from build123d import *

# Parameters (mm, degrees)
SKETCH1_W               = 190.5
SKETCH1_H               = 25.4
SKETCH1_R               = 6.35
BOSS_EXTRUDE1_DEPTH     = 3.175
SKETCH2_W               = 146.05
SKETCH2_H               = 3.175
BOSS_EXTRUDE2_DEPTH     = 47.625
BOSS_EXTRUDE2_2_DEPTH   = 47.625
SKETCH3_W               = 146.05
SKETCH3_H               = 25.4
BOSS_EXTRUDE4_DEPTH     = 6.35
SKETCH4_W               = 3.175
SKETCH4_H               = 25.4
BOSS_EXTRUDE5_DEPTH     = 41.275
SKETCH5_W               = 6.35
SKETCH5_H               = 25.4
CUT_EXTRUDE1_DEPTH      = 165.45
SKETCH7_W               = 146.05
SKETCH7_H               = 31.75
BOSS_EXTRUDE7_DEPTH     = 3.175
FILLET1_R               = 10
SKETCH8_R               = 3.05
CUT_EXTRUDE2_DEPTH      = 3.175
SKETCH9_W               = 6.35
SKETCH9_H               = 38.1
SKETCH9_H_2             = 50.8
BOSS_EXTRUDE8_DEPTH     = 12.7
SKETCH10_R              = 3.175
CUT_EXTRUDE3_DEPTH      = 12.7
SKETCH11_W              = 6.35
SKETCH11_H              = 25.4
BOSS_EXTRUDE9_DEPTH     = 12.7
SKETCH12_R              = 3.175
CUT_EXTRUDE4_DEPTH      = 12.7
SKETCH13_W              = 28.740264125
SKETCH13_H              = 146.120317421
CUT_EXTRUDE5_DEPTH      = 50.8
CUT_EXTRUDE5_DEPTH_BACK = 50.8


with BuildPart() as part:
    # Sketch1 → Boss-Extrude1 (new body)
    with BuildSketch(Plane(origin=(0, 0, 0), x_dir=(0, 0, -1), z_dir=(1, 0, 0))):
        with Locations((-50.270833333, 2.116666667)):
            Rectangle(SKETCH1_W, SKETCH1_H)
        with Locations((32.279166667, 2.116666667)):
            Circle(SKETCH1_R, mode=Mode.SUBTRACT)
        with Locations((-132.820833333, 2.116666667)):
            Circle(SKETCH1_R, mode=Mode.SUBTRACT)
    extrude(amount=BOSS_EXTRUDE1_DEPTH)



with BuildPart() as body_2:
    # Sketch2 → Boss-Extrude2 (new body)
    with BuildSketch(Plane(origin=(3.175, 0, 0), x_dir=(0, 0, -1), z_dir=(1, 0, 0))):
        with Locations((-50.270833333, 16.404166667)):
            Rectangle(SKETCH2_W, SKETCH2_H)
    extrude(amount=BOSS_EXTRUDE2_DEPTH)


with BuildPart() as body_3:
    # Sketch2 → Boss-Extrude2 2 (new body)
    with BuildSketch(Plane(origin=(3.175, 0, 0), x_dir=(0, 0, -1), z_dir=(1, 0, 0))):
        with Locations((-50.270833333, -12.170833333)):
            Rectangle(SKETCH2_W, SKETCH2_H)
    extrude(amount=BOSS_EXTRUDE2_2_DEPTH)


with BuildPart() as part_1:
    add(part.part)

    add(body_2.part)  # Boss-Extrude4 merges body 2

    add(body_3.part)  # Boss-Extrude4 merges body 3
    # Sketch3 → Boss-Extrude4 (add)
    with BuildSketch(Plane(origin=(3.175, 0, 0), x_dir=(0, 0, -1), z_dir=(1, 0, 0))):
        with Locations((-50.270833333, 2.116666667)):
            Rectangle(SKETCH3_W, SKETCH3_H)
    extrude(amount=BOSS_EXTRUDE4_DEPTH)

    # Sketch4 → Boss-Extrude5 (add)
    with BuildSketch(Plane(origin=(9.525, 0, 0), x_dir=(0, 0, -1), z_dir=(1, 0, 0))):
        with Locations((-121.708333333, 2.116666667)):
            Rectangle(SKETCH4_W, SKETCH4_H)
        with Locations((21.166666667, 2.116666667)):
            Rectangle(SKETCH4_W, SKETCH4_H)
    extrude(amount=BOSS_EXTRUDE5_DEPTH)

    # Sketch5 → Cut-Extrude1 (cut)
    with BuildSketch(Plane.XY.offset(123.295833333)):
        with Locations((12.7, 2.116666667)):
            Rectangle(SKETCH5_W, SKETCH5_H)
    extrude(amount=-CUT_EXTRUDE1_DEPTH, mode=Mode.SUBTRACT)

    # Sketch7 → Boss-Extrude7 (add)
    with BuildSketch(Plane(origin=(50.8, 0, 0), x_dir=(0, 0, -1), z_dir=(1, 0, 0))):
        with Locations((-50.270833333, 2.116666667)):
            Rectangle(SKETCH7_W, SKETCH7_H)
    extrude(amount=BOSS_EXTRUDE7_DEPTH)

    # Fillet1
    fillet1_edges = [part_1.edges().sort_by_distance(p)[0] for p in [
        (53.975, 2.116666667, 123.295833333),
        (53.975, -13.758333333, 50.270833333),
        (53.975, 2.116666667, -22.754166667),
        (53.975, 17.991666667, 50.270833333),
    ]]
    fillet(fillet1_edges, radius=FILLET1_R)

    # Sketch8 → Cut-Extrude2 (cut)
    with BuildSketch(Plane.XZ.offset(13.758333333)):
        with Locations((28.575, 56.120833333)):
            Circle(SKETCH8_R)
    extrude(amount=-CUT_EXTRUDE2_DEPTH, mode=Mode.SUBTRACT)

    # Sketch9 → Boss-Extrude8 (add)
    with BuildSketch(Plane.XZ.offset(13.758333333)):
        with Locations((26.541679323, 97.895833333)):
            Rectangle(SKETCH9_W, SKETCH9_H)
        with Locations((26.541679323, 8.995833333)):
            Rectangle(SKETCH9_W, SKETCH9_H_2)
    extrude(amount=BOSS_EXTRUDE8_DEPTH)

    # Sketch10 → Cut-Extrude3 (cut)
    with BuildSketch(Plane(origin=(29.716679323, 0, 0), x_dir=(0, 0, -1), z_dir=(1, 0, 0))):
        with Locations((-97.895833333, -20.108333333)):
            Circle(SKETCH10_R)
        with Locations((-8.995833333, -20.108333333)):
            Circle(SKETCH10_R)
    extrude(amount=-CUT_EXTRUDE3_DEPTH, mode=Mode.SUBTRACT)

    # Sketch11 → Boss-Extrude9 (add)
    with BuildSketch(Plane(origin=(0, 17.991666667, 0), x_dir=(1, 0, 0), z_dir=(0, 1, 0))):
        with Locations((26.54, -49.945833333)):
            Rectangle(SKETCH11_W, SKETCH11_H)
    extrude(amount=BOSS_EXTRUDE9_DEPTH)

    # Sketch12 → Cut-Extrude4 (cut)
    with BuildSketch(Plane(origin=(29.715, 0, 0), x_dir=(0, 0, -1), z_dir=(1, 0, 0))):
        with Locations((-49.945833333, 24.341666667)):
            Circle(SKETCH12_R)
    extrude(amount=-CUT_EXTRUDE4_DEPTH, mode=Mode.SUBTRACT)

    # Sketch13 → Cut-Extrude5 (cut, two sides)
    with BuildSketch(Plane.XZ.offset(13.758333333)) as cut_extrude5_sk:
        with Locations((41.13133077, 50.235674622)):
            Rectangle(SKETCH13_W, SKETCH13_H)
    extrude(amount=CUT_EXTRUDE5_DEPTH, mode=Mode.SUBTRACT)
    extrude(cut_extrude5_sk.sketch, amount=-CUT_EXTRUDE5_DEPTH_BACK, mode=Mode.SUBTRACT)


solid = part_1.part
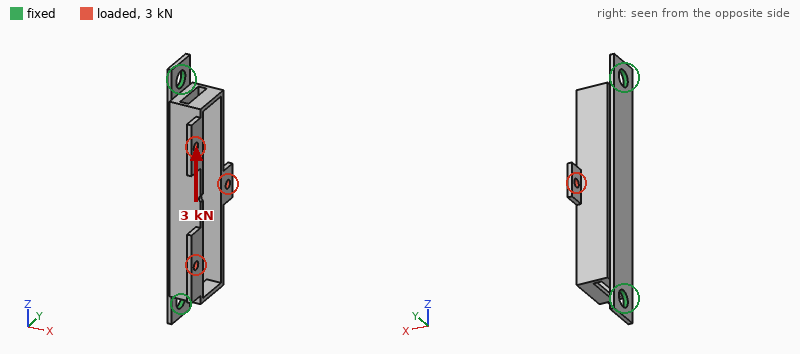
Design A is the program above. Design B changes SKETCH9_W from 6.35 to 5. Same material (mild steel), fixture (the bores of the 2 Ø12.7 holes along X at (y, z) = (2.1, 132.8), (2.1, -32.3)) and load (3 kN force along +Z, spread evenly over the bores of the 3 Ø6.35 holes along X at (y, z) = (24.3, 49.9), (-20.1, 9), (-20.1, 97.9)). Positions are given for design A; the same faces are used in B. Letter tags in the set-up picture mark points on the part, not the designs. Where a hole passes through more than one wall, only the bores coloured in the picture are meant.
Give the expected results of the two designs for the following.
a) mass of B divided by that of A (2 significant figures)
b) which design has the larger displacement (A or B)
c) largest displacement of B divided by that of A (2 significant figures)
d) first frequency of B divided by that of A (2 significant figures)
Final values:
0.99
B
1.1
1.0
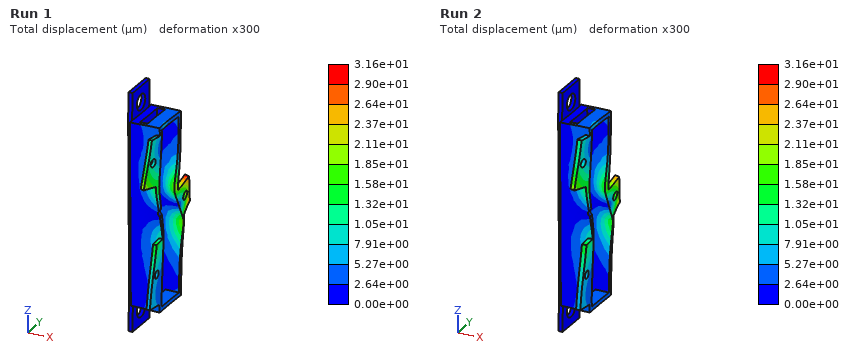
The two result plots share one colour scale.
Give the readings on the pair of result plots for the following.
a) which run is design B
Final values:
Run 1
